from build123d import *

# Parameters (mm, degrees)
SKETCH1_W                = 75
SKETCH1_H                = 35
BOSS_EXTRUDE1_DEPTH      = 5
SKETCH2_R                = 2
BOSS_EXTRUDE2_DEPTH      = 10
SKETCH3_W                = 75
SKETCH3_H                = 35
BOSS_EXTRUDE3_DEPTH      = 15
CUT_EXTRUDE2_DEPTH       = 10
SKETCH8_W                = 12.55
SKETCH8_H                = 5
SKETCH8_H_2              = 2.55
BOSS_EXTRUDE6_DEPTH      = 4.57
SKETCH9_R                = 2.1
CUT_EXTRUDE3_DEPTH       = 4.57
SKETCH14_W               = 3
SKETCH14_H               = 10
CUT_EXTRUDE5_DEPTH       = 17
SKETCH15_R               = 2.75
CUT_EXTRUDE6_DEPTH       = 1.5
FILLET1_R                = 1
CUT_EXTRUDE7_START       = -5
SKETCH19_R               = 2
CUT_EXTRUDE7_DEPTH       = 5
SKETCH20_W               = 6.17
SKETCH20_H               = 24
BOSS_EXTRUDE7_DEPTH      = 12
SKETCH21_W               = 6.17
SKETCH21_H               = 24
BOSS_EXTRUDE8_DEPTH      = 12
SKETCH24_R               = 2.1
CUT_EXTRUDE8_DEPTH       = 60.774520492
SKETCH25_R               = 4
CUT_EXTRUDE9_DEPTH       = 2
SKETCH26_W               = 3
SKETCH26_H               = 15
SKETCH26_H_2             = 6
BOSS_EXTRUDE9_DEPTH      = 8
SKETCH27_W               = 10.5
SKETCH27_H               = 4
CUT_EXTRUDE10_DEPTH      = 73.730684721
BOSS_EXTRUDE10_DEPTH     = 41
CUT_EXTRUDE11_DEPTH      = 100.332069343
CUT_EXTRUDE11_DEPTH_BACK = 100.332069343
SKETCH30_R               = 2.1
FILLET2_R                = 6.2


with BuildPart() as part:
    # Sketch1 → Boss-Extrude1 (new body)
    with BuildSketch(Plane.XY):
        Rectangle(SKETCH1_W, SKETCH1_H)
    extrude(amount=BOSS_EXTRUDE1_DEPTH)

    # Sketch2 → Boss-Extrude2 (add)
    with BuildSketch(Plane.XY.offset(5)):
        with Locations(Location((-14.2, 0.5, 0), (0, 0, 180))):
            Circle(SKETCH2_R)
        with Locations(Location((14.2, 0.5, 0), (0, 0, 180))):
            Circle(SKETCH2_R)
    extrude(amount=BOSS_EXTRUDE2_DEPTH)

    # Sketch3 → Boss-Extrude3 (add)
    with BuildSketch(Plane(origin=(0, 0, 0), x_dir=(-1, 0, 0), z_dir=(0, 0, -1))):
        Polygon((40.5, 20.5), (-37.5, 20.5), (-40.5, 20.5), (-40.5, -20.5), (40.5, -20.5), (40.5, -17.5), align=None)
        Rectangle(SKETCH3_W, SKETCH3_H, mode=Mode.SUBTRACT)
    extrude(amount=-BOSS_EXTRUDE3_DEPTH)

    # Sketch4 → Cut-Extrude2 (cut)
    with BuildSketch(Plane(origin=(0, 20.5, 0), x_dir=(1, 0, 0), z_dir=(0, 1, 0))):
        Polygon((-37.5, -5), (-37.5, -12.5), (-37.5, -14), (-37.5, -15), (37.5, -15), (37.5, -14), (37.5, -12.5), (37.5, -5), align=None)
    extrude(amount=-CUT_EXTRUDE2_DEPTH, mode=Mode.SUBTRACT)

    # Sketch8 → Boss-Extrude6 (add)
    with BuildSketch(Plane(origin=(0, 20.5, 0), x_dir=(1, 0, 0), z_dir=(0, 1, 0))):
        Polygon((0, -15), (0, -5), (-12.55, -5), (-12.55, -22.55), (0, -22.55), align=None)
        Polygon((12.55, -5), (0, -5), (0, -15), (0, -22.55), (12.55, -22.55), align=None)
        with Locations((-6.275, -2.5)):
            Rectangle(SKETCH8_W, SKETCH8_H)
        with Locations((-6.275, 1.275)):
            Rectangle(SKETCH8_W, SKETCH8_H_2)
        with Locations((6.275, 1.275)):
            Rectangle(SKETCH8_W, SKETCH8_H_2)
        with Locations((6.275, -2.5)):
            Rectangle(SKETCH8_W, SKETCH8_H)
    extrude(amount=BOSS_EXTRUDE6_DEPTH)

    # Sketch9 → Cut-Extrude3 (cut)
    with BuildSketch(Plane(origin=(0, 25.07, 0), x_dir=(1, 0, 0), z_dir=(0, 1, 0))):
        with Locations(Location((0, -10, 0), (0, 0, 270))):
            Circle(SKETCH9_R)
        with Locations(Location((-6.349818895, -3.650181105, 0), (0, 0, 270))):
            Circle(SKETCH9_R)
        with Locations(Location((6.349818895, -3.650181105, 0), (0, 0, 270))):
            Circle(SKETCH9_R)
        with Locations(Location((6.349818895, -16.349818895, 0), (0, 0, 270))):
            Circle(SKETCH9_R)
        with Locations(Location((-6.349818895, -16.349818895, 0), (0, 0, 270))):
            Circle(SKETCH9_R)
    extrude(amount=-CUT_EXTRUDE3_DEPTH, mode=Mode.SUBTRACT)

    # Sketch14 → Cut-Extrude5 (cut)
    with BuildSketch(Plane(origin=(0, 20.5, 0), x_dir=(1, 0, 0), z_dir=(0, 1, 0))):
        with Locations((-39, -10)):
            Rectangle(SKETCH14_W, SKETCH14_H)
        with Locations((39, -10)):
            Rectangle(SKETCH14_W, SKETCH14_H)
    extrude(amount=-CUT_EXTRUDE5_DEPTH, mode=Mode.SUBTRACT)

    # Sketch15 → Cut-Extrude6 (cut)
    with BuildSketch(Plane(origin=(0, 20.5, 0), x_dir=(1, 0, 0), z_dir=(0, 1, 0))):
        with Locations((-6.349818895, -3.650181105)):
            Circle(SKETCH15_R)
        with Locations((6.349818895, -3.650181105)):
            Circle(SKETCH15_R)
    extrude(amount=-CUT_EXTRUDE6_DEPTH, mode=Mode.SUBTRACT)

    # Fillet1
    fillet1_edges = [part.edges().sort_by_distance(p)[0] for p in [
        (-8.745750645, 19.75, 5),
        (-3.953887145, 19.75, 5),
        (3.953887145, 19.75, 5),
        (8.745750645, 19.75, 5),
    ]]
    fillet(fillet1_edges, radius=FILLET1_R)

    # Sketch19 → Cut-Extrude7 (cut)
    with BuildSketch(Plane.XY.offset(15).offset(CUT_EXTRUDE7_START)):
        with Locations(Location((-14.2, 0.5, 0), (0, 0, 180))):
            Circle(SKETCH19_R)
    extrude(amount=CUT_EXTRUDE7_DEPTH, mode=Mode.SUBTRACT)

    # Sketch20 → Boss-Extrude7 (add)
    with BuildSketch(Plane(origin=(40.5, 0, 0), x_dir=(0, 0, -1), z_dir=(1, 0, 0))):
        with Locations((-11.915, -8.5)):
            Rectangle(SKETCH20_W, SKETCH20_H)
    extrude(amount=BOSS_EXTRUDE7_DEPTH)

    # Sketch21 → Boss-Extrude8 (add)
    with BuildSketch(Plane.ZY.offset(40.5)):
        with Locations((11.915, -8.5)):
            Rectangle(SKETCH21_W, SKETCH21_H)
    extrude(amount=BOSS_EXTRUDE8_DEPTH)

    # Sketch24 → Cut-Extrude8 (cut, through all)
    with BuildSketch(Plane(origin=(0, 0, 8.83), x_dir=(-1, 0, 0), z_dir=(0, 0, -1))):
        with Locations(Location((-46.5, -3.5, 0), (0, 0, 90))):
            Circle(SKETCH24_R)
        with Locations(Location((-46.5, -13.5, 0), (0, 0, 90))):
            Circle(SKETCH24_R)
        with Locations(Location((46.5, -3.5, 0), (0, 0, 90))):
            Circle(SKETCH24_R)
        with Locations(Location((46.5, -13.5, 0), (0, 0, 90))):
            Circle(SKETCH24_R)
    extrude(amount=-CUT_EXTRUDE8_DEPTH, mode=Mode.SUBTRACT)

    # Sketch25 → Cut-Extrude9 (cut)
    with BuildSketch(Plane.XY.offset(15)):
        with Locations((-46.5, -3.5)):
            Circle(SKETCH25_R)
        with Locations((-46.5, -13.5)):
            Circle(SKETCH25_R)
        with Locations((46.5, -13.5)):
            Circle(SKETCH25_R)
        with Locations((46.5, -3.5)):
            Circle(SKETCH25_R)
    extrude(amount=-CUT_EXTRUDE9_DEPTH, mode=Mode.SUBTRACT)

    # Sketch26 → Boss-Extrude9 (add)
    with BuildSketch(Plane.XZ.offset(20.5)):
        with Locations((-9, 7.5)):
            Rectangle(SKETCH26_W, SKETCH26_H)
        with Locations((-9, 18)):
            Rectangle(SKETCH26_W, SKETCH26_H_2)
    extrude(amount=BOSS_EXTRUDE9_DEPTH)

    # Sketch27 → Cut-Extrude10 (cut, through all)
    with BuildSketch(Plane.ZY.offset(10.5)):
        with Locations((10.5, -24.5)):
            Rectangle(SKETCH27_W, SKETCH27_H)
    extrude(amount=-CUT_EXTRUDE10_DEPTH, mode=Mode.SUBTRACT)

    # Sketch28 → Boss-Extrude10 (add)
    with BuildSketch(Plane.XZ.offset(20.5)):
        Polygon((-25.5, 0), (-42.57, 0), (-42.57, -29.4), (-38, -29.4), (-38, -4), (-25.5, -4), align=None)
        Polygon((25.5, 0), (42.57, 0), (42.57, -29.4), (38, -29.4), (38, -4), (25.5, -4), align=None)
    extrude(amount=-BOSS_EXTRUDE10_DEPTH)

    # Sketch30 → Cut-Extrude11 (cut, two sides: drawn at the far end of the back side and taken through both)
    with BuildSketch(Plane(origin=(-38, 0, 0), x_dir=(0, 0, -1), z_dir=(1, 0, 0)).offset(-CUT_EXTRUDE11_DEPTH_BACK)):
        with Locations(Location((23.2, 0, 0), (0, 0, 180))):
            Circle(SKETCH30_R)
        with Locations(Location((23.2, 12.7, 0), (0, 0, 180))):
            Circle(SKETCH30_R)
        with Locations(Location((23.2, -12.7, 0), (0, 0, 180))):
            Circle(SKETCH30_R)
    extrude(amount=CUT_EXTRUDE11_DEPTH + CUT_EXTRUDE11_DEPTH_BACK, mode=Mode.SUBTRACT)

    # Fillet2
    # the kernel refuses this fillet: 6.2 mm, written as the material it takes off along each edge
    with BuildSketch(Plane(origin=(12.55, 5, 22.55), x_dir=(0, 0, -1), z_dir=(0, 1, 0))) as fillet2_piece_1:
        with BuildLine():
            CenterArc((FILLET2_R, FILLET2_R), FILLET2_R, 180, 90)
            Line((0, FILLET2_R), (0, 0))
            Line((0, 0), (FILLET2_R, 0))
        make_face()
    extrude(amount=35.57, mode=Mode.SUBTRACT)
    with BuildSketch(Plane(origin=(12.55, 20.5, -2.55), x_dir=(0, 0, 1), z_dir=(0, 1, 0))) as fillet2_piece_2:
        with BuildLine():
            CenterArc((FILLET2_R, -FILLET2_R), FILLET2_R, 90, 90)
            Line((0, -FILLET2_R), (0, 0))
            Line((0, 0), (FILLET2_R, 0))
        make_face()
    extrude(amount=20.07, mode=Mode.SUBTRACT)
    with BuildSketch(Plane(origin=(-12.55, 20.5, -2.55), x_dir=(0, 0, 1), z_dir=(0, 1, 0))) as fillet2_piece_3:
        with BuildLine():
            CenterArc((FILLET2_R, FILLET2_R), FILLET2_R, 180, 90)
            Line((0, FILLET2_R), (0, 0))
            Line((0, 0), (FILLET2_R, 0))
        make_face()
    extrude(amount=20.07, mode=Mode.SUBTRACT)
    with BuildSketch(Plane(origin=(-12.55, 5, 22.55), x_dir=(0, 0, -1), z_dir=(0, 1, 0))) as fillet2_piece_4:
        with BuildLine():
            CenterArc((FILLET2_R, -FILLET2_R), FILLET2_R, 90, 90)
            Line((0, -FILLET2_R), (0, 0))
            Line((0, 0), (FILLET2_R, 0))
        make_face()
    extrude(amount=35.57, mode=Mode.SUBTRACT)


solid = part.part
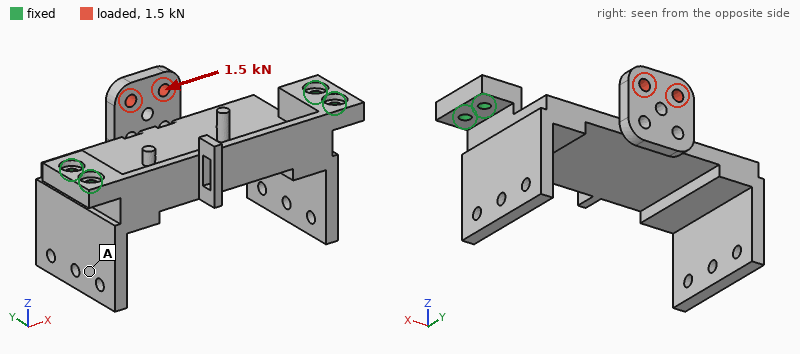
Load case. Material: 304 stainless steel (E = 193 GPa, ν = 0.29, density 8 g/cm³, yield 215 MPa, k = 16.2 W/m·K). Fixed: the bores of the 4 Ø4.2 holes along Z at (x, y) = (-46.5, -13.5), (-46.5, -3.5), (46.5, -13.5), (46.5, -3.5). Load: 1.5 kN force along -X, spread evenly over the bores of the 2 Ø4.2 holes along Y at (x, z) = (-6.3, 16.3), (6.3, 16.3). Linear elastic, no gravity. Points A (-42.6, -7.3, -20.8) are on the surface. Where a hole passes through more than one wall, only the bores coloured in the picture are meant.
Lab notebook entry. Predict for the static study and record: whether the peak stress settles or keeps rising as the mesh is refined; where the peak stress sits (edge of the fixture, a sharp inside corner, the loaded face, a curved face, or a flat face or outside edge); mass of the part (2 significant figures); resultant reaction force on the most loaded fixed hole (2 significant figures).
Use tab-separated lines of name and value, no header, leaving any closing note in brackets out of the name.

whether the peak stress settles or keeps rising as the mesh is refined	keeps rising
where the peak stress sits	a sharp inside corner
mass of the part	330 g
resultant reaction force on the most loaded fixed hole	1.2 kN
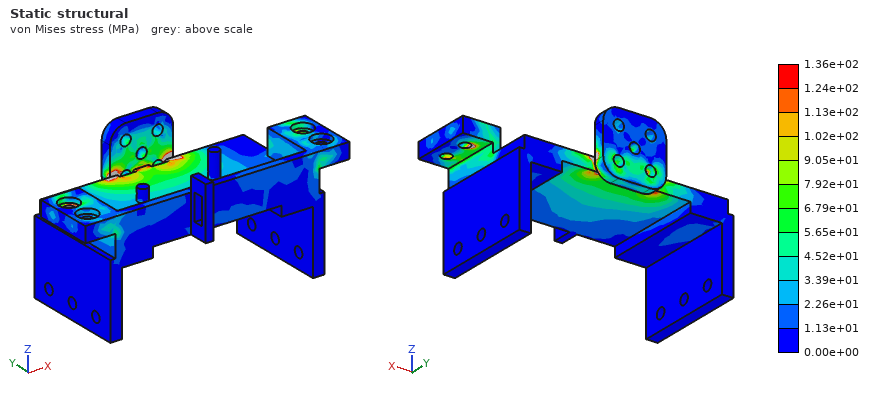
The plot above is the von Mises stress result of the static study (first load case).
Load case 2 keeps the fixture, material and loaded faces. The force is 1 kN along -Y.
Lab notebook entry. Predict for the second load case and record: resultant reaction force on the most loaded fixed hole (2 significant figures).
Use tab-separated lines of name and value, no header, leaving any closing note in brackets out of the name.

resultant reaction force on the most loaded fixed hole	340 N
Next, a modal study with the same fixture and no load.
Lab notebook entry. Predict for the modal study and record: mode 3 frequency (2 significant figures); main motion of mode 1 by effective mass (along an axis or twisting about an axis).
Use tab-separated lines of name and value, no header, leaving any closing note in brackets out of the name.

mode 3 frequency	3000 Hz
main motion of mode 1 by effective mass	along Z
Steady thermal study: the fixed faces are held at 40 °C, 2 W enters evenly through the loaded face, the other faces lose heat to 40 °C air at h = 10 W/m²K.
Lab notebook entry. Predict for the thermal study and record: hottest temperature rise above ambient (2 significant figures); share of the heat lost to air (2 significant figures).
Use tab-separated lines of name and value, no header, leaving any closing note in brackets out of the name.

hottest temperature rise above ambient	34 K
share of the heat lost to air	59 %
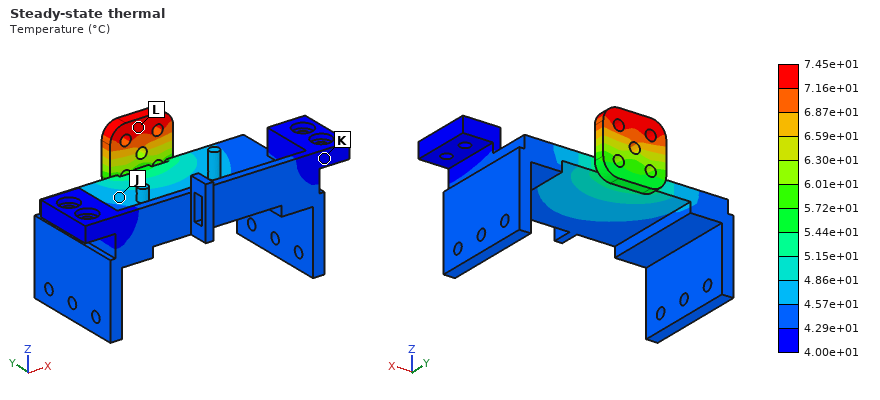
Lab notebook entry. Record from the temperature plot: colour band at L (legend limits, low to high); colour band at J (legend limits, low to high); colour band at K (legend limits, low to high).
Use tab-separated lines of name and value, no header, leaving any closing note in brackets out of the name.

colour band at L	7.16e+01 to 7.45e+01 °C
colour band at J	4.57e+01 to 4.86e+01 °C
colour band at K	4.00e+01 to 4.29e+01 °C
